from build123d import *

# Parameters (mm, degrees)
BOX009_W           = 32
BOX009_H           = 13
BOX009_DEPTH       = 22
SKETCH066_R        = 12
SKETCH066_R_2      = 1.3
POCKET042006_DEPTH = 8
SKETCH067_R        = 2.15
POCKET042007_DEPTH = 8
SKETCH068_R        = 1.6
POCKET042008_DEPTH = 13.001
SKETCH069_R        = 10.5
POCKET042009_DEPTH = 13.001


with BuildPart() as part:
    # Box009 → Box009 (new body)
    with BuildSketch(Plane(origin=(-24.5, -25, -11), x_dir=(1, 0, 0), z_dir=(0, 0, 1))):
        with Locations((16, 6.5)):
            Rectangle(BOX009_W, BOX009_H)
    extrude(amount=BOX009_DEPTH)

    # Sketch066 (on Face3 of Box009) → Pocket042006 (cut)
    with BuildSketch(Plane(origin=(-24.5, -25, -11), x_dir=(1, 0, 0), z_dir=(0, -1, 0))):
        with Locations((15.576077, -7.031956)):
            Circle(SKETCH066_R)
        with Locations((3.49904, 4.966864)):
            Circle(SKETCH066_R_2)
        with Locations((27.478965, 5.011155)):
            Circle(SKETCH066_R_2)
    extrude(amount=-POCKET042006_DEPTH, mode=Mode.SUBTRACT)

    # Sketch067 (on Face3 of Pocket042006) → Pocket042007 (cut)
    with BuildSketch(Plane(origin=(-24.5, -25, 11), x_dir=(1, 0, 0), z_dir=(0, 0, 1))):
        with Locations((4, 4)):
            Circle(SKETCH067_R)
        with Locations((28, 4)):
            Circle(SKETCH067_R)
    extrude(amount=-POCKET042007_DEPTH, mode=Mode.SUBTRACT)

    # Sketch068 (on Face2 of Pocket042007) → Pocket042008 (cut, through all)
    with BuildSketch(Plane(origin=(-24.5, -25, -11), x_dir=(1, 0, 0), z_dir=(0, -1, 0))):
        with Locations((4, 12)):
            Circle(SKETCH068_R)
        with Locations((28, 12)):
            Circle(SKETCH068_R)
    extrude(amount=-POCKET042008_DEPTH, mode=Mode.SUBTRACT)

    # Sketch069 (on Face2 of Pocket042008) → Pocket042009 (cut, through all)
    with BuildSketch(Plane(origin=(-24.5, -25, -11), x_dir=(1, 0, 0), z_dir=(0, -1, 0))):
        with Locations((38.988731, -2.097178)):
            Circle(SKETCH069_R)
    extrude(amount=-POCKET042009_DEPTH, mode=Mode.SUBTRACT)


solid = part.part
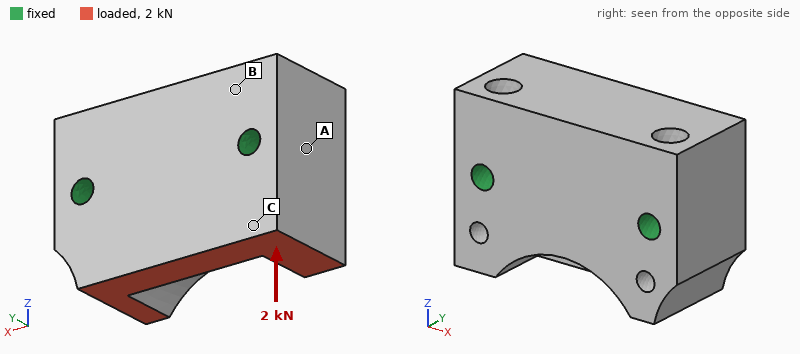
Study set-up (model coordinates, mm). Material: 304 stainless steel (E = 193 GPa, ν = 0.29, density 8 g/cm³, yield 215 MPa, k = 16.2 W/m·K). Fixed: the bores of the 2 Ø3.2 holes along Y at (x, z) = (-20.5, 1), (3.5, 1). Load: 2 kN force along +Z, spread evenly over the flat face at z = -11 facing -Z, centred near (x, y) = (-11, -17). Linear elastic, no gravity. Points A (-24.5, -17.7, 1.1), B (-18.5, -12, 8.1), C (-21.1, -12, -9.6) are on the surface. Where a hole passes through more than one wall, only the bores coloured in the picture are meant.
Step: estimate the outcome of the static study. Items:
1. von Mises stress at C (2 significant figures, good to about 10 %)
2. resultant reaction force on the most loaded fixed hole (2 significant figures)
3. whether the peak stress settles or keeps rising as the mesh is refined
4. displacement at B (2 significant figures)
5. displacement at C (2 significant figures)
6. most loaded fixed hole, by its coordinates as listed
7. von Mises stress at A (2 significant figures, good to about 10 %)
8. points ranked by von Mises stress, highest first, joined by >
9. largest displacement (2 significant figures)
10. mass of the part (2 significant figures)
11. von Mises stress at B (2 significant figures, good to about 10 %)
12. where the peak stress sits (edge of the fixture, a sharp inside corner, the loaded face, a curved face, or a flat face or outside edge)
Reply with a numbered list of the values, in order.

1. 9.2 MPa
2. 1.2 kN
3. keeps rising
4. 0.21 µm
5. 0.71 µm
6. (-20.5, 1)
7. 5.3 MPa
8. C > A > B
9. 1.1 µm
10. 63 g
11. 2.8 MPa
12. edge of the fixture
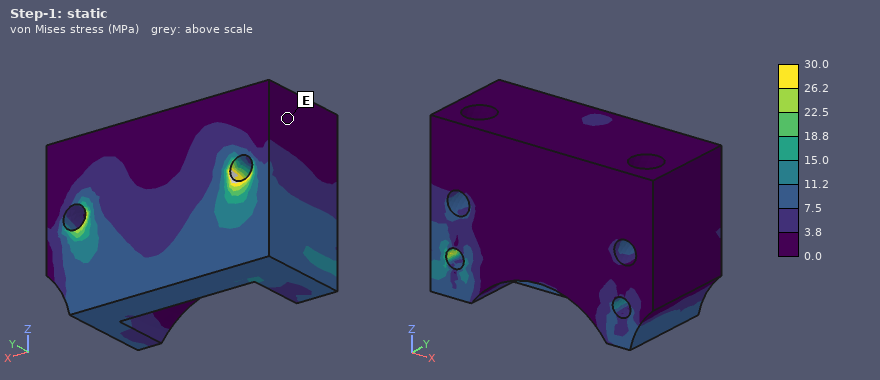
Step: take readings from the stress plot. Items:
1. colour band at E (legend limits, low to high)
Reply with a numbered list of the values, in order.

1. 0.0 to 3.8 MPa
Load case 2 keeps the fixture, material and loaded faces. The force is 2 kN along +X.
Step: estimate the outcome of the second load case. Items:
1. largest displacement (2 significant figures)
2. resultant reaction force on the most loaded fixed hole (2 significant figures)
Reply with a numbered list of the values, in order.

1. 2.7 µm
2. 1.4 kN
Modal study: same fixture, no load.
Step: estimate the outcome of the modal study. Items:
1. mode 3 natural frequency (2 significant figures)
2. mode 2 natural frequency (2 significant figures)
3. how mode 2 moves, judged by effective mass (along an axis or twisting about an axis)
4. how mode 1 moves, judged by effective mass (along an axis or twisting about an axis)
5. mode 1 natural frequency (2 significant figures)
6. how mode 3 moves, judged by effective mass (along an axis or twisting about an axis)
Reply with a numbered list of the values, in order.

1. 45 kHz
2. 39 kHz
3. along Y
4. twisting about X
5. 36 kHz
6. along Z
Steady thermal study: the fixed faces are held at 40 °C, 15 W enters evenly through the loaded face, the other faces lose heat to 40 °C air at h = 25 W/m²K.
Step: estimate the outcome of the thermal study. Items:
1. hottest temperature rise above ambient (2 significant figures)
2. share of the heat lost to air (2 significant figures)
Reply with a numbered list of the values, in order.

1. 45 K
2. 5.4 %
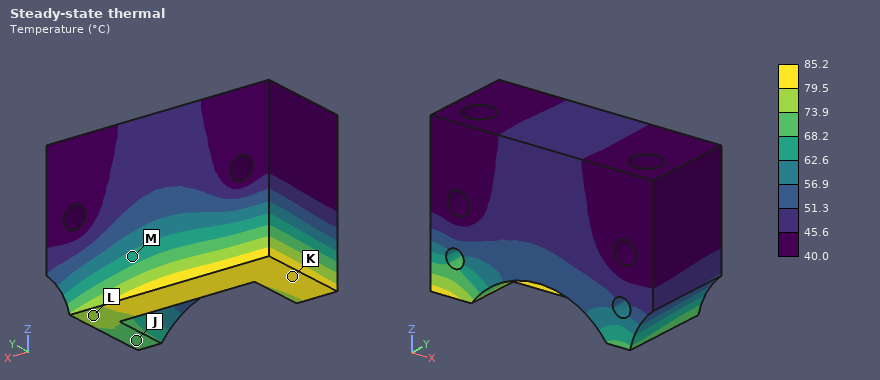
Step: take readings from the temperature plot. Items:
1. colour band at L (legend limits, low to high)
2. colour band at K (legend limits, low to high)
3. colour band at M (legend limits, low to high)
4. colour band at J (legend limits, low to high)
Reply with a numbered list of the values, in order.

1. 73.9 to 79.5 °C
2. 79.5 to 85.2 °C
3. 62.6 to 68.2 °C
4. 68.2 to 73.9 °C
